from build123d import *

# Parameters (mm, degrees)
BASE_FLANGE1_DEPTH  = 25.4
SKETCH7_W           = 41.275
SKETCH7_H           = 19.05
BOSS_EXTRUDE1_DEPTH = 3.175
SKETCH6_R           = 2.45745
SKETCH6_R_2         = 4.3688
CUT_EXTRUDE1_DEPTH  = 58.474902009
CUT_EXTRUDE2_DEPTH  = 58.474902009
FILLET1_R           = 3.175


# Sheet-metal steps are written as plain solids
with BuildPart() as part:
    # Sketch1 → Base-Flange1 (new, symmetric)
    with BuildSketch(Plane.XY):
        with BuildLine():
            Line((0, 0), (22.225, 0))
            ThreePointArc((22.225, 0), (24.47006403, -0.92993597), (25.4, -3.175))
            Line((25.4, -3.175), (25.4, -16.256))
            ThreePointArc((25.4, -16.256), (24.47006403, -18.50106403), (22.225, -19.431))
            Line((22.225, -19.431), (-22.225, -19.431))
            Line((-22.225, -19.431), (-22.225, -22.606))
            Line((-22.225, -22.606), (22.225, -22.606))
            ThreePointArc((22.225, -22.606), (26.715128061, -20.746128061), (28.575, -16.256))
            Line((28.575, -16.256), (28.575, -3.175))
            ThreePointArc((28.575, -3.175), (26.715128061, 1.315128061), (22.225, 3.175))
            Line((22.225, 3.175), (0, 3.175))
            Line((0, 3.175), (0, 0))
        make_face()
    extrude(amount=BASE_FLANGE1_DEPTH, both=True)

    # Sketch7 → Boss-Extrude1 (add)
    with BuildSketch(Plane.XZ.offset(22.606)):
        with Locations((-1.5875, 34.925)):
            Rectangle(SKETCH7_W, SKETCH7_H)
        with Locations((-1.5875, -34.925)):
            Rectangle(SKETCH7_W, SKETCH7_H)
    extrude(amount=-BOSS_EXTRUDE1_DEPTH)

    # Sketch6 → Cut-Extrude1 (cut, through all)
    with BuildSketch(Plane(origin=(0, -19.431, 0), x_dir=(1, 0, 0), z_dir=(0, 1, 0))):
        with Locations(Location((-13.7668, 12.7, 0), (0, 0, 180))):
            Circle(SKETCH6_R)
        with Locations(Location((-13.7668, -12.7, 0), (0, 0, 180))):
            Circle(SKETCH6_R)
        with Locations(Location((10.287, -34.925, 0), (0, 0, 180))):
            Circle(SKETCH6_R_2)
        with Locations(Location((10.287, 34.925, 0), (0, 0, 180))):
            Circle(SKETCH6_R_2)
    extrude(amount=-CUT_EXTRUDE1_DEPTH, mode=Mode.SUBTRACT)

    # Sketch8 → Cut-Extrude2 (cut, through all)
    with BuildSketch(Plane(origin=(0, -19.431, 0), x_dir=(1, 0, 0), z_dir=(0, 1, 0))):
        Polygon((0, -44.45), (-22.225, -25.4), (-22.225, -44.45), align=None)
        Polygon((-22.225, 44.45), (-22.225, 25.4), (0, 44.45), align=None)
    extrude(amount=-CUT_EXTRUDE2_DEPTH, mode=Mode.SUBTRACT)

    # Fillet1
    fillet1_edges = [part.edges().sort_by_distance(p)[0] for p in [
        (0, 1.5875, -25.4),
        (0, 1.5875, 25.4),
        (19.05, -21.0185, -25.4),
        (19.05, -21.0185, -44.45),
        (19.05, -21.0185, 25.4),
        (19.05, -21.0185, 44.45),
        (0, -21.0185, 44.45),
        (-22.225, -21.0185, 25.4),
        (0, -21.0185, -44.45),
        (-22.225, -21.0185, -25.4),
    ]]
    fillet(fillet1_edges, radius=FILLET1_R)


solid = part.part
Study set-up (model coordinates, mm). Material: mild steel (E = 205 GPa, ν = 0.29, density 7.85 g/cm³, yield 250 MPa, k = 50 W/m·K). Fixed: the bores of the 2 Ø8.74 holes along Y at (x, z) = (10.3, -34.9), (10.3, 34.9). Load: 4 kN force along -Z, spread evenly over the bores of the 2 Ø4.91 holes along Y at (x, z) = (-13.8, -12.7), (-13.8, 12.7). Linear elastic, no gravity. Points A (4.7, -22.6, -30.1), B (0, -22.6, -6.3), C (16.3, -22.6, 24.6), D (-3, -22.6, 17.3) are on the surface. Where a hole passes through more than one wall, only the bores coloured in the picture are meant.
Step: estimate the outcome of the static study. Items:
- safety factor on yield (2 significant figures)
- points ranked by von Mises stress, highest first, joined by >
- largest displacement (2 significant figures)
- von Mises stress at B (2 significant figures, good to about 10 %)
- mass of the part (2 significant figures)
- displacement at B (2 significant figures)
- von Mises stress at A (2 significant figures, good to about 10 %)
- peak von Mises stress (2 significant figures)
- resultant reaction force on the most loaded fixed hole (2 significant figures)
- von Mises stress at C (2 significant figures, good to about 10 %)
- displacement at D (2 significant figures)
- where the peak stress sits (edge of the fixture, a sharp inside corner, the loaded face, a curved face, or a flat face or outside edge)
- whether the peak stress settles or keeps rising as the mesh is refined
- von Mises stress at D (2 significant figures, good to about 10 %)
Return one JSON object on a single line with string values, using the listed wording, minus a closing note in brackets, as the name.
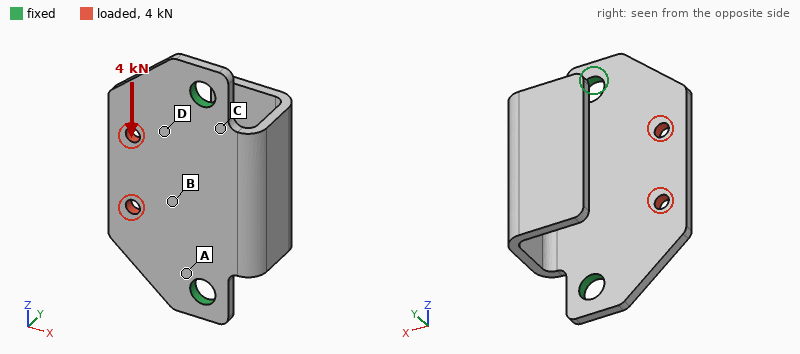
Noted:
{"safety factor on yield": "2.8", "points ranked by von Mises stress, highest first, joined by >": "A > D > B > C", "largest displacement": "7.8 µm", "von Mises stress at B": "25 MPa", "mass of the part": "140 g", "displacement at B": "3.5 µm", "von Mises stress at A": "45 MPa", "peak von Mises stress": "89 MPa", "resultant reaction force on the most loaded fixed hole": "2.4 kN", "von Mises stress at C": "14 MPa", "displacement at D": "3.7 µm", "where the peak stress sits": "the loaded face", "whether the peak stress settles or keeps rising as the mesh is refined": "settles", "von Mises stress at D": "33 MPa"}
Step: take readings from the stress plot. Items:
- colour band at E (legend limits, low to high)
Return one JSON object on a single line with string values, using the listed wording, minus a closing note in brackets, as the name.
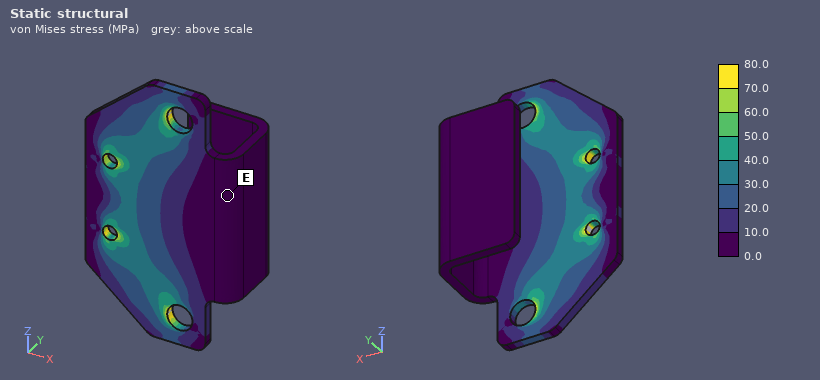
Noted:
{"colour band at E": "0.0 to 10.0 MPa"}
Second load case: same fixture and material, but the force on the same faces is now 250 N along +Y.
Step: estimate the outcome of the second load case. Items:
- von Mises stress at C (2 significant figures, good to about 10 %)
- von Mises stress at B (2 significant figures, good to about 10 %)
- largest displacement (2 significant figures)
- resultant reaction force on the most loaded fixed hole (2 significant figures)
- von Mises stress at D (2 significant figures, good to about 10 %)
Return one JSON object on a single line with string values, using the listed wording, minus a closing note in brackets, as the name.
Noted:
{"von Mises stress at C": "28 MPa", "von Mises stress at B": "23 MPa", "largest displacement": "78 µm", "resultant reaction force on the most loaded fixed hole": "130 N", "von Mises stress at D": "25 MPa"}
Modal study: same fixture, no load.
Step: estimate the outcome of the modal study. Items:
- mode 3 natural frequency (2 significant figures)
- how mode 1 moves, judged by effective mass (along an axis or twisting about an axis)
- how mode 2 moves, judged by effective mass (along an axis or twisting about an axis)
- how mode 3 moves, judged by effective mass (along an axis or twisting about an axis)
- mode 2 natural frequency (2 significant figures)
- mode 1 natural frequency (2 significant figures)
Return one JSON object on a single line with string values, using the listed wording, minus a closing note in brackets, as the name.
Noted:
{"mode 3 natural frequency": "2000 Hz", "how mode 1 moves, judged by effective mass": "along X", "how mode 2 moves, judged by effective mass": "along Z", "how mode 3 moves, judged by effective mass": "along Y", "mode 2 natural frequency": "1800 Hz", "mode 1 natural frequency": "1000 Hz"}
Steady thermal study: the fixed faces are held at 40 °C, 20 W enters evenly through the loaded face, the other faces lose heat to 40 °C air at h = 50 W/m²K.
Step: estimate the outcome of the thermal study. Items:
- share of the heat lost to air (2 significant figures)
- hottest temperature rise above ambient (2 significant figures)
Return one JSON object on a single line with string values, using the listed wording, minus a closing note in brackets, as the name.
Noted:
{"share of the heat lost to air": "45 %", "hottest temperature rise above ambient": "56 K"}
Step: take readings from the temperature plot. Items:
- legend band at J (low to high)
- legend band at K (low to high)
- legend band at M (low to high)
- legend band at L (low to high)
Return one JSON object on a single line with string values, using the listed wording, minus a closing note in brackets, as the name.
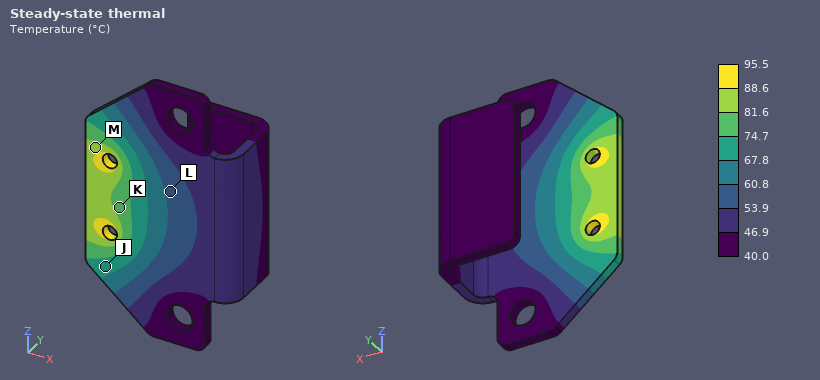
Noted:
{"legend band at J": "67.8 to 74.7 °C", "legend band at K": "74.7 to 81.6 °C", "legend band at M": "81.6 to 88.6 °C", "legend band at L": "53.9 to 60.8 °C"}
